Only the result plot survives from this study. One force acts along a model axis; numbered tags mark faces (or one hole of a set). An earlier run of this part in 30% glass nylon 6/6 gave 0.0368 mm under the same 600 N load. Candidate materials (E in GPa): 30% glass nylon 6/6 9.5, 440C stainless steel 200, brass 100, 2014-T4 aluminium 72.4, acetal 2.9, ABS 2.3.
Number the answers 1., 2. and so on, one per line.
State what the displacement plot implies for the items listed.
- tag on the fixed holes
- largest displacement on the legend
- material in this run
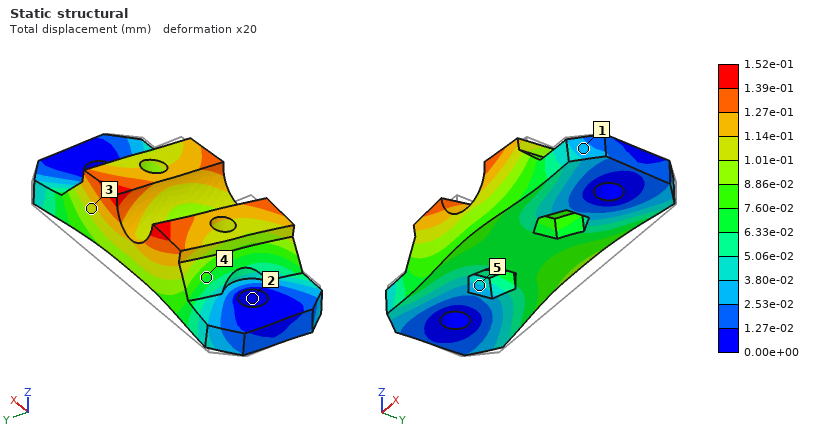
1. 2
2. 1.52e-01 mm
3. ABS
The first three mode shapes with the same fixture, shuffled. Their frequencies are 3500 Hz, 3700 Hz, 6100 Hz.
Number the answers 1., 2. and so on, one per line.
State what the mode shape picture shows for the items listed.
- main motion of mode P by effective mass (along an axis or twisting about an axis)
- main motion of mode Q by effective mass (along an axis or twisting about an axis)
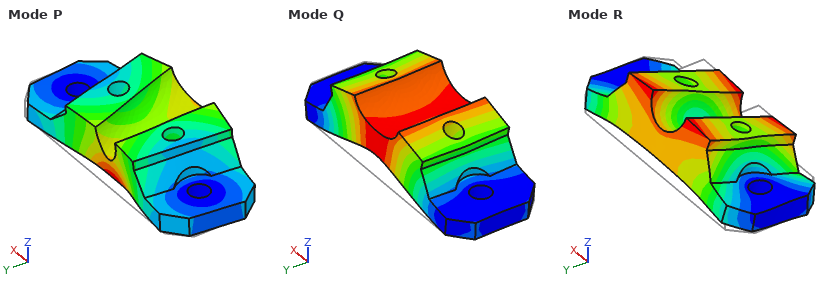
1. along Y
2. along Z
